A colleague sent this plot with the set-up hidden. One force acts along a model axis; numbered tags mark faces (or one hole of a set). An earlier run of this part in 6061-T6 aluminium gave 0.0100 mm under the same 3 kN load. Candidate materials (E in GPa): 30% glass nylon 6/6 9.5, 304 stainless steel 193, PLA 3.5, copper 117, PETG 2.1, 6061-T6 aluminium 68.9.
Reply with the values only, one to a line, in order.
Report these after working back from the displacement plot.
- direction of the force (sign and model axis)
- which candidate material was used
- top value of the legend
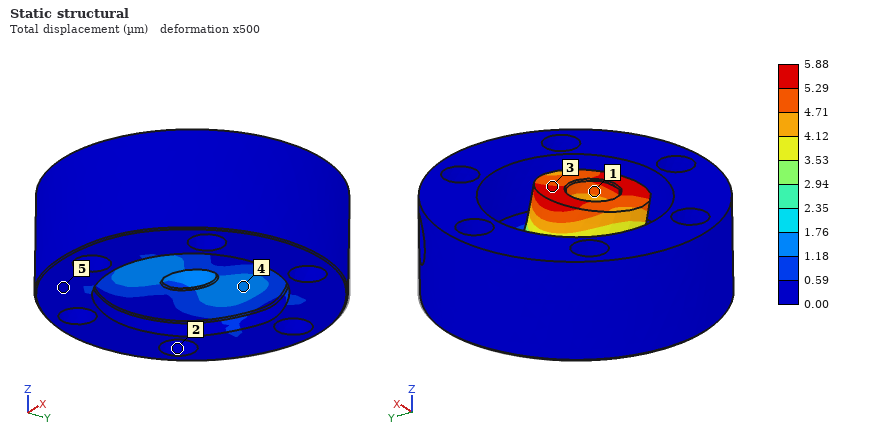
-Y
copper
5.88 µm
